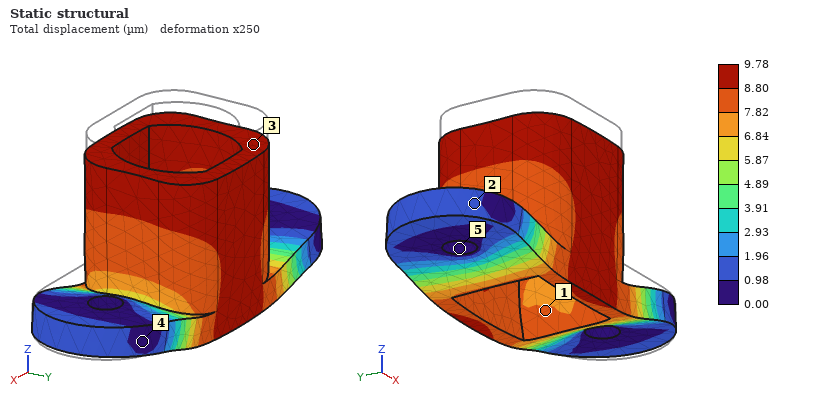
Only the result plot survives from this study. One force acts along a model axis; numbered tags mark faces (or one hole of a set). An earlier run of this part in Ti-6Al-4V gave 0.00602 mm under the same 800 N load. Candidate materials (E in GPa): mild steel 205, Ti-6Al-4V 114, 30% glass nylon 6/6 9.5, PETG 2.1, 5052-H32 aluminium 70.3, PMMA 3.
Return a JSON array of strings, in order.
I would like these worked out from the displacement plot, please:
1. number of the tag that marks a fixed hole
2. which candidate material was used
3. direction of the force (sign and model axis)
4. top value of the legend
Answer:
["5", "5052-H32 aluminium", "-Z", "9.78 µm"]
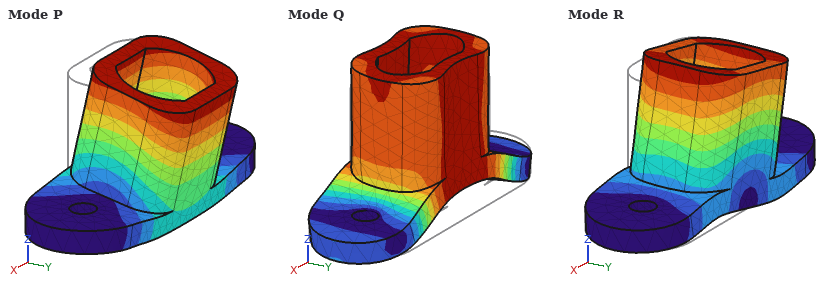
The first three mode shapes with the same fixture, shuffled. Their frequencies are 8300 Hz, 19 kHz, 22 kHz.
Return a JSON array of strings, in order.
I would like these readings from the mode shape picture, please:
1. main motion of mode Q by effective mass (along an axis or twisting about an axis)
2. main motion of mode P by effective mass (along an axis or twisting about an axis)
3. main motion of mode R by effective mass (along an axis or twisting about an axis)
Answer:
["along Z", "along Y", "along X"]
